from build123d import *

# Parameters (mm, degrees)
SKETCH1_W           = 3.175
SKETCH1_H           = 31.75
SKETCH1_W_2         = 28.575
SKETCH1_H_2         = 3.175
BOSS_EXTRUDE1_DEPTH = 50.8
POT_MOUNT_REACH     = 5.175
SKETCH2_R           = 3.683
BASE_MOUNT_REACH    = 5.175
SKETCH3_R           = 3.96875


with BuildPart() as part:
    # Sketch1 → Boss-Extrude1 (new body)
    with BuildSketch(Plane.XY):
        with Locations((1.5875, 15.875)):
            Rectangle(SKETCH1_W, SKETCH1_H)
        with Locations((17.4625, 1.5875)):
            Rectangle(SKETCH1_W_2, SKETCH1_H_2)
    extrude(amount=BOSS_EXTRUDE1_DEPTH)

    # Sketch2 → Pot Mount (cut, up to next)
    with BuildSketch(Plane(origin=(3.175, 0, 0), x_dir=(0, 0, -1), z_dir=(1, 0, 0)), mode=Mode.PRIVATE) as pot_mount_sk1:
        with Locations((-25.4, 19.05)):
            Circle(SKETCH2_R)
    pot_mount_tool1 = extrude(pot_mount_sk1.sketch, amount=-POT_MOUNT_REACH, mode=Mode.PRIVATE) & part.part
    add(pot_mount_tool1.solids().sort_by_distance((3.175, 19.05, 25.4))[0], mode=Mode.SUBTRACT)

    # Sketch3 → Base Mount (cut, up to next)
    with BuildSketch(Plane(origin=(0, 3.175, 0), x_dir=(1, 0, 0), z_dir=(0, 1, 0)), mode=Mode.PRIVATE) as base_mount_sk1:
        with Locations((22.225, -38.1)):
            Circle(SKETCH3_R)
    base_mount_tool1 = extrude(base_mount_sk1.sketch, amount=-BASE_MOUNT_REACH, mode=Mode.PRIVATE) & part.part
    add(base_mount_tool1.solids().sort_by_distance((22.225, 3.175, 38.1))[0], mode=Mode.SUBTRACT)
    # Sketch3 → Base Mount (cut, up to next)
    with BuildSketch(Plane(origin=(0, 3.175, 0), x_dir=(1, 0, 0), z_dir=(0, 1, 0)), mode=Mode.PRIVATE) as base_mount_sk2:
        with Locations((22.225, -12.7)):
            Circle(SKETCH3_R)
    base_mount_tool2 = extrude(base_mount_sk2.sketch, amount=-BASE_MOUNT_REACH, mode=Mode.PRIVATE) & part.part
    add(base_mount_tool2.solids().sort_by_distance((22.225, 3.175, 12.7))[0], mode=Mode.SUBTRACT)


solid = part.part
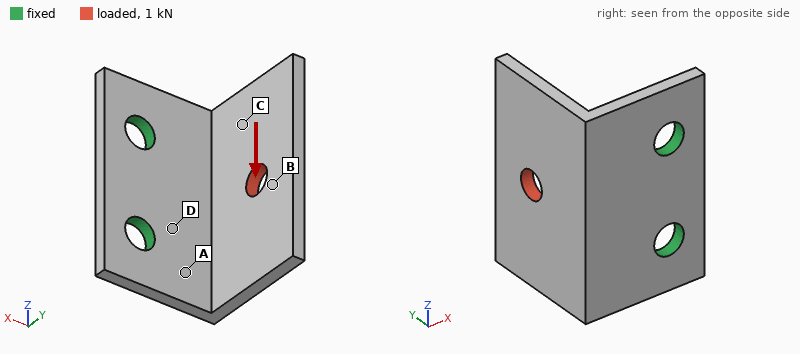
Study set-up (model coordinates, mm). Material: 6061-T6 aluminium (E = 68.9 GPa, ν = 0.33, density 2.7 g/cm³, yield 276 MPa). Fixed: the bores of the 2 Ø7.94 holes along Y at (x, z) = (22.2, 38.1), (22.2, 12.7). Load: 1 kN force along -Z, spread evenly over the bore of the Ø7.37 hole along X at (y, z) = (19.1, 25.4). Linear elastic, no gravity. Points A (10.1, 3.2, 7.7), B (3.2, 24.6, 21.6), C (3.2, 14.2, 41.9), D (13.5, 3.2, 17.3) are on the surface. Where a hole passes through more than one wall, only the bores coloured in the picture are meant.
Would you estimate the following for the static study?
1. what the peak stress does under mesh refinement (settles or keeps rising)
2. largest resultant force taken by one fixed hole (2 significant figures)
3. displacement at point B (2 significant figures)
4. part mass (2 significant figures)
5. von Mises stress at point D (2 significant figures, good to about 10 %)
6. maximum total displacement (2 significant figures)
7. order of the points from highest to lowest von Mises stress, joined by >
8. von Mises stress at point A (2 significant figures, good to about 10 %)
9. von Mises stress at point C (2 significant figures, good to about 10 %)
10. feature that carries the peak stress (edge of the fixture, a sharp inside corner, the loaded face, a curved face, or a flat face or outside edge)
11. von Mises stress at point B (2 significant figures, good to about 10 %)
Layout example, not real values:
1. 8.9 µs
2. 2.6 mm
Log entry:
1. keeps rising
2. 940 N
3. 0.19 mm
4. 25 g
5. 85 MPa
6. 0.33 mm
7. D > A > C > B
8. 59 MPa
9. 38 MPa
10. edge of the fixture
11. 17 MPa
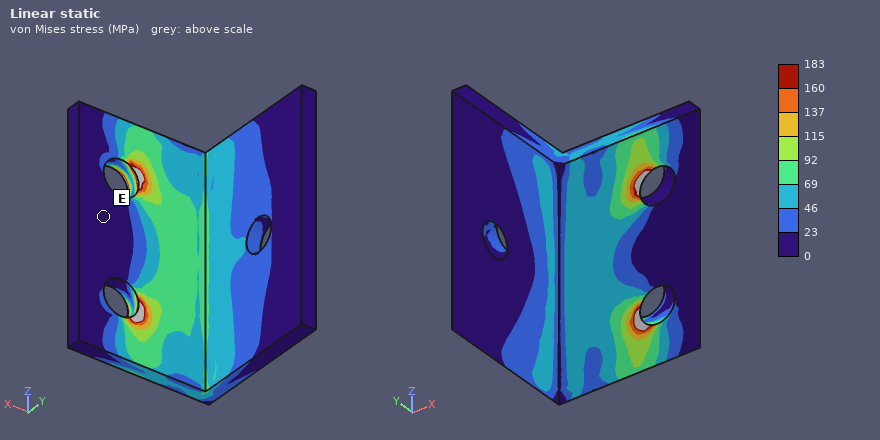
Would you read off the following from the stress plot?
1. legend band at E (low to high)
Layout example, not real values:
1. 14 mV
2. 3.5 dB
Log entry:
1. 0 to 23 MPa
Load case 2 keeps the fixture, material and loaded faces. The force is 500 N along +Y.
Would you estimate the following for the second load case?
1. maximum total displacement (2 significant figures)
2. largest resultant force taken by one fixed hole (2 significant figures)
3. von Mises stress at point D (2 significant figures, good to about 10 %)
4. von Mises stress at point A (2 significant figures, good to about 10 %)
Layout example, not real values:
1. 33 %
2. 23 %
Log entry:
1. 0.29 mm
2. 250 N
3. 66 MPa
4. 45 MPa
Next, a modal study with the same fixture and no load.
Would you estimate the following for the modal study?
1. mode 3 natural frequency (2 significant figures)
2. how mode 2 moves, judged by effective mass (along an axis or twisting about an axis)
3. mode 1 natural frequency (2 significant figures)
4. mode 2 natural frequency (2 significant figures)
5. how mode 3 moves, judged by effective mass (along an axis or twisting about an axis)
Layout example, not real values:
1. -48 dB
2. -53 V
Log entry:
1. 4400 Hz
2. along Z
3. 1500 Hz
4. 2700 Hz
5. along Y
